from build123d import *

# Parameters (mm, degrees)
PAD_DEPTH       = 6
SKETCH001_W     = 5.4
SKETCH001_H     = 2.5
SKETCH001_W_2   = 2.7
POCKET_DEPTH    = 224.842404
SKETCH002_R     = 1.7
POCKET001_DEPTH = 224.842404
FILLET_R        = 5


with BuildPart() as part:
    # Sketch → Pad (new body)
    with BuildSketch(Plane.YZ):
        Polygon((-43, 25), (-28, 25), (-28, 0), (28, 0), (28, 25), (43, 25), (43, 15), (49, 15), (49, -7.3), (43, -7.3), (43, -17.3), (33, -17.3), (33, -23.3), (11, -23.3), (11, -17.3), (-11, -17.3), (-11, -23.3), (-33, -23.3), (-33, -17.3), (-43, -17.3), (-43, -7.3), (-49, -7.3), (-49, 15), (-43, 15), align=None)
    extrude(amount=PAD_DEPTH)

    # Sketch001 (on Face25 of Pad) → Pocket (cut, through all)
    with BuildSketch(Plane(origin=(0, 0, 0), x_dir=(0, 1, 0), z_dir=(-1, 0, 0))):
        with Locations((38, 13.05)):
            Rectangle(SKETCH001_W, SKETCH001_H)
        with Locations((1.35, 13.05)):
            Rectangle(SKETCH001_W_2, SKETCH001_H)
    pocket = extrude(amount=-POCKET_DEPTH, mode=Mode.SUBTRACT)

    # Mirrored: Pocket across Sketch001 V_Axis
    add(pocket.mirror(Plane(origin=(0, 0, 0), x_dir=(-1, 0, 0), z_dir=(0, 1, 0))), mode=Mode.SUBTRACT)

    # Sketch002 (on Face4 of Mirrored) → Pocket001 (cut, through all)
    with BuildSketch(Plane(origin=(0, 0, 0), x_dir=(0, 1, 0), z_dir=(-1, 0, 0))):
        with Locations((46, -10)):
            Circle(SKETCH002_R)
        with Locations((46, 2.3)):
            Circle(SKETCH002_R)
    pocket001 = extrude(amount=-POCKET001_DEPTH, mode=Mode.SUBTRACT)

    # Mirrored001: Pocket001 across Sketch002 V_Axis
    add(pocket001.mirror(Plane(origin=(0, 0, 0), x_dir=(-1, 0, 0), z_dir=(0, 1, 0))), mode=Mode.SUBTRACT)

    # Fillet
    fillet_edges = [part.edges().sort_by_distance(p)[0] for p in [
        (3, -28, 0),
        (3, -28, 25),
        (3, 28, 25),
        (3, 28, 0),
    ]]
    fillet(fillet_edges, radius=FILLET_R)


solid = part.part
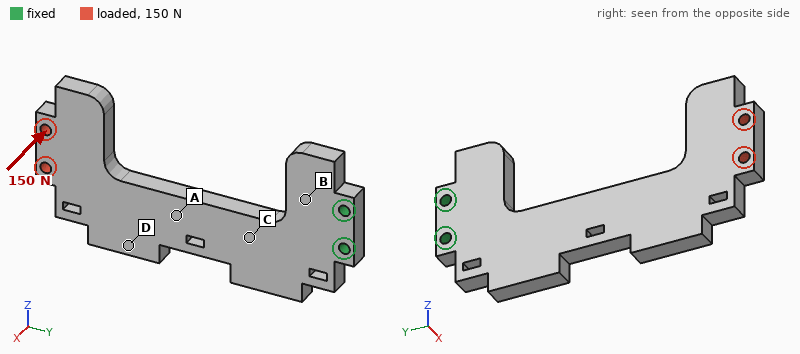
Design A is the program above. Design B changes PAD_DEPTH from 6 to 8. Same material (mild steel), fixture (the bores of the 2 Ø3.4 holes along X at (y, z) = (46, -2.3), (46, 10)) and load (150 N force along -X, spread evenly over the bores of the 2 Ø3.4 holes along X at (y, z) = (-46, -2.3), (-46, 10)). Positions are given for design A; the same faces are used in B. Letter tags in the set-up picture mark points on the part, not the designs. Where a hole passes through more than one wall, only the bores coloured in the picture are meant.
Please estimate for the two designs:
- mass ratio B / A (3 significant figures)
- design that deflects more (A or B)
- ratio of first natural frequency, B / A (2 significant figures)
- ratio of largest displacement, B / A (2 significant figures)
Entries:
1.33
A
1.3
0.44
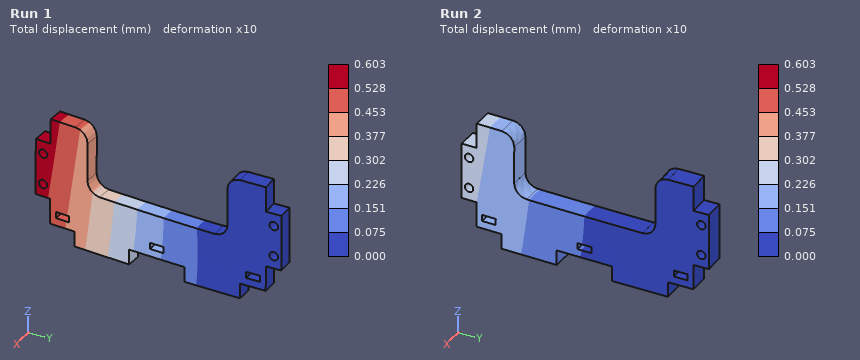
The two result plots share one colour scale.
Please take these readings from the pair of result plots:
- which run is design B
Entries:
Run 2
